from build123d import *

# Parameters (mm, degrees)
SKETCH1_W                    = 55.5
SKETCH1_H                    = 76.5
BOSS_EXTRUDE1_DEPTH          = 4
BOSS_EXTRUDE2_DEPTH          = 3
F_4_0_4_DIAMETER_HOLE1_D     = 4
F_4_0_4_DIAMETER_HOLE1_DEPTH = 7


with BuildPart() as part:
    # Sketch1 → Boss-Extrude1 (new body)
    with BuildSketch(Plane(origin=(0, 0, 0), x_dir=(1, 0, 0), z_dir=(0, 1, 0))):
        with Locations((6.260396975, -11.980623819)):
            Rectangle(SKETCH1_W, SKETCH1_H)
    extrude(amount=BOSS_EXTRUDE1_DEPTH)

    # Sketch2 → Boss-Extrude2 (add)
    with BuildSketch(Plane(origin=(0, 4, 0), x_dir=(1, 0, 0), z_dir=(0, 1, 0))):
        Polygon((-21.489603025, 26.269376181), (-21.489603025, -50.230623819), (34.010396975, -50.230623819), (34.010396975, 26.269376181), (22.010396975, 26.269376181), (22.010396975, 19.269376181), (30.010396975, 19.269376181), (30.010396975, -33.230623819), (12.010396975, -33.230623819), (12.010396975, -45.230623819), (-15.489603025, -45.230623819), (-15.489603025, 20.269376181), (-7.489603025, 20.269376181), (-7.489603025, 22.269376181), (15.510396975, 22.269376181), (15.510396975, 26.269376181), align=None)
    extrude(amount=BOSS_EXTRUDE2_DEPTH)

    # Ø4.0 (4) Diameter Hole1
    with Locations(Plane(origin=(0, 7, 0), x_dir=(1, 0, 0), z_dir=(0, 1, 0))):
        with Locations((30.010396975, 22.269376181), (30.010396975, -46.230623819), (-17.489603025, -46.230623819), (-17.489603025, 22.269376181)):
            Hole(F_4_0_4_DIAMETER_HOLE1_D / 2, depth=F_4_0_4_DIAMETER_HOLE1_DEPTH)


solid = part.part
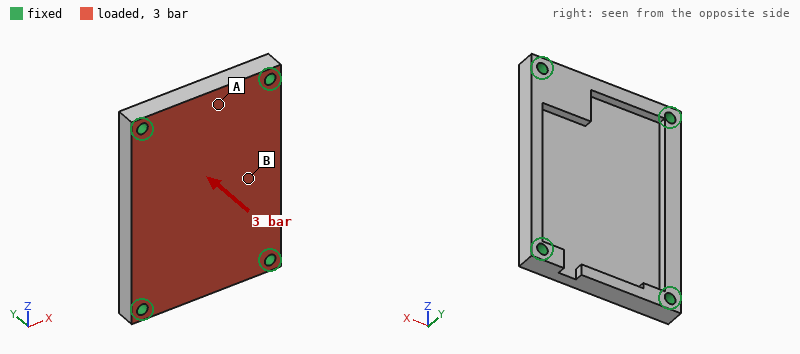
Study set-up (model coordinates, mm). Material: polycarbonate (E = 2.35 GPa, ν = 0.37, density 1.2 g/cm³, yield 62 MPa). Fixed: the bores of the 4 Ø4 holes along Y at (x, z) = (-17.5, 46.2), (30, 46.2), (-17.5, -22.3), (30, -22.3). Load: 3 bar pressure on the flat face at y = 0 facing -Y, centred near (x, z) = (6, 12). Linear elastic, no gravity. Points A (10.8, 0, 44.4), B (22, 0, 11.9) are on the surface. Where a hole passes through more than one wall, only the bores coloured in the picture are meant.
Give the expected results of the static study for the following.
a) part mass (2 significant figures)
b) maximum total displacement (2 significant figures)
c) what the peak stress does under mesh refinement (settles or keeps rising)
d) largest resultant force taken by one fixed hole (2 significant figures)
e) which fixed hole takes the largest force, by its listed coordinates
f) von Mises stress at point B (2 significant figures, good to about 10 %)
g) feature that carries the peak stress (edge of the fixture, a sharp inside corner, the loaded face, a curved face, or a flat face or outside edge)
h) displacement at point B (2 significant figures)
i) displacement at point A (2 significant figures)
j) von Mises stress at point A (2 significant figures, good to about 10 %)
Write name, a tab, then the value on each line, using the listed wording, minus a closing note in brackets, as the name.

part mass	25 g
maximum total displacement	1.1 mm
what the peak stress does under mesh refinement	keeps rising
largest resultant force taken by one fixed hole	410 N
which fixed hole takes the largest force, by its listed coordinates	(30, 46.2)
von Mises stress at point B	14 MPa
feature that carries the peak stress	edge of the fixture
displacement at point B	0.87 mm
displacement at point A	0.22 mm
von Mises stress at point A	6.8 MPa
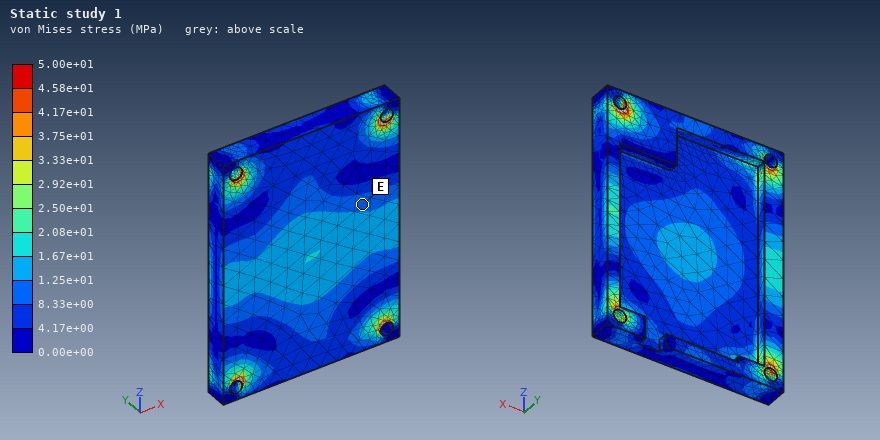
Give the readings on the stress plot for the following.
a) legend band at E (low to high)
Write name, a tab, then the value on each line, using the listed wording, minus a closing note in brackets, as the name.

legend band at E	8.33e+00 to 1.25e+01 MPa
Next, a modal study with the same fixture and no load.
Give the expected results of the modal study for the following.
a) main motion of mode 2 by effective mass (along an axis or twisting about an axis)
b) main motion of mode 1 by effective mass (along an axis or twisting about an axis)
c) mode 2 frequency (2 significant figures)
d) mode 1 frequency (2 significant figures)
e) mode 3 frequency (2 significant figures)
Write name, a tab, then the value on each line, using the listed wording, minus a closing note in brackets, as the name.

main motion of mode 2 by effective mass	twisting about Z
main motion of mode 1 by effective mass	along Y
mode 2 frequency	2100 Hz
mode 1 frequency	1400 Hz
mode 3 frequency	3000 Hz
